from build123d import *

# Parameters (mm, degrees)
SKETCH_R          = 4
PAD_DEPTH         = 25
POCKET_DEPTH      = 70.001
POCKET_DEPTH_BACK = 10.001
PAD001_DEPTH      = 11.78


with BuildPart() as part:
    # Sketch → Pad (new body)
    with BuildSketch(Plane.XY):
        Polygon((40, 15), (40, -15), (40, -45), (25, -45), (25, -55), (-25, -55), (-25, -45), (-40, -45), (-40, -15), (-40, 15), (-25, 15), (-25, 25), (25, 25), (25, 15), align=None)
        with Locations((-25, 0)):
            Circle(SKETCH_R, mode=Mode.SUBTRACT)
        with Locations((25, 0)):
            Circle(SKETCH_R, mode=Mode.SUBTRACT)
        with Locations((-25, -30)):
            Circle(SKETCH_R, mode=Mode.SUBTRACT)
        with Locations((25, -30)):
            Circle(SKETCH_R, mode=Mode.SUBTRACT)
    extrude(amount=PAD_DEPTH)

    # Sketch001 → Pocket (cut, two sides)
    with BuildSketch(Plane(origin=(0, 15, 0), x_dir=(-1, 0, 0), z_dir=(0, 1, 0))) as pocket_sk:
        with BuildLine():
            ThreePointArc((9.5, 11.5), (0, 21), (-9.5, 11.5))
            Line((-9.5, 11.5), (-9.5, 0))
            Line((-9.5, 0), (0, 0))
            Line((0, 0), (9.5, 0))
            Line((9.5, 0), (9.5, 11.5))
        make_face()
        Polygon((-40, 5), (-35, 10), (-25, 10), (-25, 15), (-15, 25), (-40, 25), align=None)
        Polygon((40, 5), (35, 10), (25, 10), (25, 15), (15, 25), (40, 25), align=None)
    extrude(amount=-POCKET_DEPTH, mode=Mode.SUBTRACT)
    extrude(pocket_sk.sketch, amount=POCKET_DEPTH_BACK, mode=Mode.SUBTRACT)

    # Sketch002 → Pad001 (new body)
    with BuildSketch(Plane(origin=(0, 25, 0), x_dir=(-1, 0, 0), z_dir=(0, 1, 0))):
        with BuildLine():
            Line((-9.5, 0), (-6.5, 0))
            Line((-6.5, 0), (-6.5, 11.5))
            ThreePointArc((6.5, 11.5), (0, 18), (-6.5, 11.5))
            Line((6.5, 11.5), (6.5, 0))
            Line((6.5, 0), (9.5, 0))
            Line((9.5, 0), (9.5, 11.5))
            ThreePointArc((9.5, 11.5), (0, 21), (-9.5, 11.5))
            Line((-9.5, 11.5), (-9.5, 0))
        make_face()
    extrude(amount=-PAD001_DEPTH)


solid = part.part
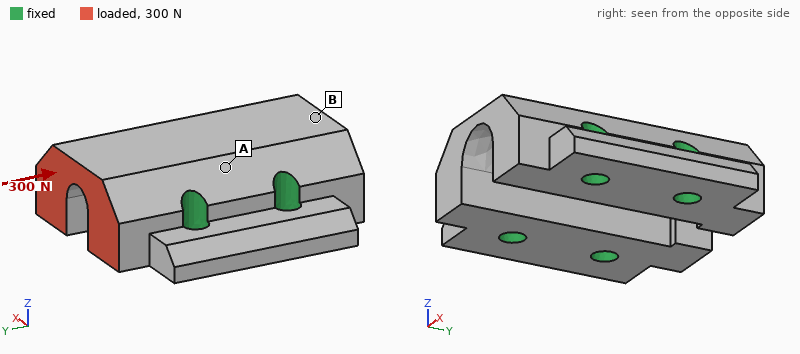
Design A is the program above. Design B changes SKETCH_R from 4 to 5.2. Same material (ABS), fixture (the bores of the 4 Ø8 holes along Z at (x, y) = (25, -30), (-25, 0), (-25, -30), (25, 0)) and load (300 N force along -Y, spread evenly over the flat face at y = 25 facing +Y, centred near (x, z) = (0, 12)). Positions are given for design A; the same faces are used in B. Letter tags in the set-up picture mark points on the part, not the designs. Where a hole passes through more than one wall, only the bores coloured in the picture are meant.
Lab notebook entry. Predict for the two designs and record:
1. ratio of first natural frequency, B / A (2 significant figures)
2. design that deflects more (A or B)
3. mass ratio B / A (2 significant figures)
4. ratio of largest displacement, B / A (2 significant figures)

1.1
A
0.98
0.90
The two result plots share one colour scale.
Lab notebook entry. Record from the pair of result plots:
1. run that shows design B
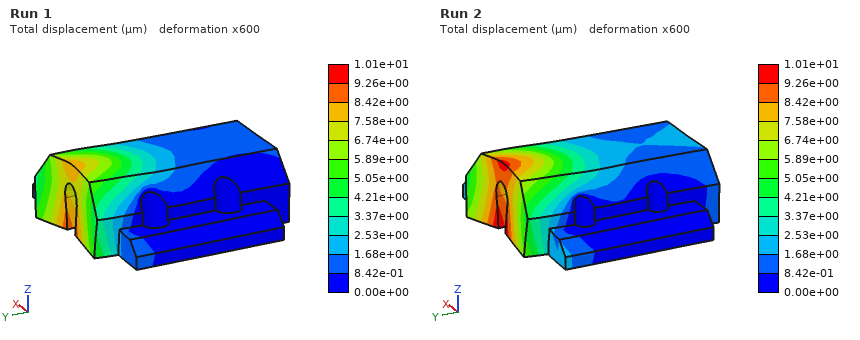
Run 1
